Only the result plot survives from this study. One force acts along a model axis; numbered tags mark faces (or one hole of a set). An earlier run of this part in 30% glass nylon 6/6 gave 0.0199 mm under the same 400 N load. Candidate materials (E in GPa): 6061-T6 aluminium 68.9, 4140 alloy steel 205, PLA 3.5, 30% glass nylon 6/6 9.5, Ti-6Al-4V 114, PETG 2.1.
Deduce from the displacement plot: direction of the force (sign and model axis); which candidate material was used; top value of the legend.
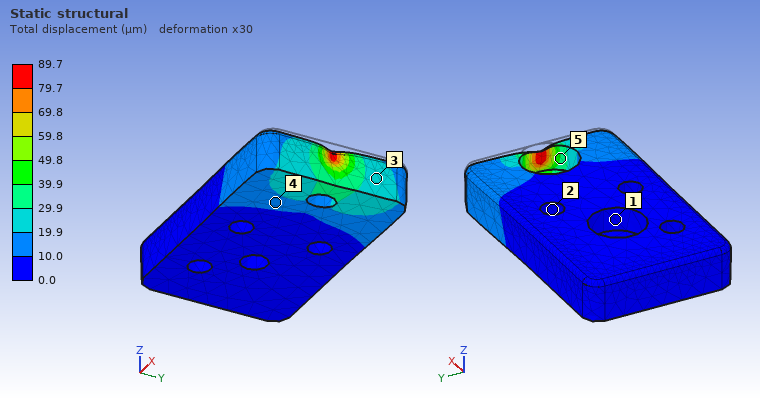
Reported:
-X
PETG
89.7 µm
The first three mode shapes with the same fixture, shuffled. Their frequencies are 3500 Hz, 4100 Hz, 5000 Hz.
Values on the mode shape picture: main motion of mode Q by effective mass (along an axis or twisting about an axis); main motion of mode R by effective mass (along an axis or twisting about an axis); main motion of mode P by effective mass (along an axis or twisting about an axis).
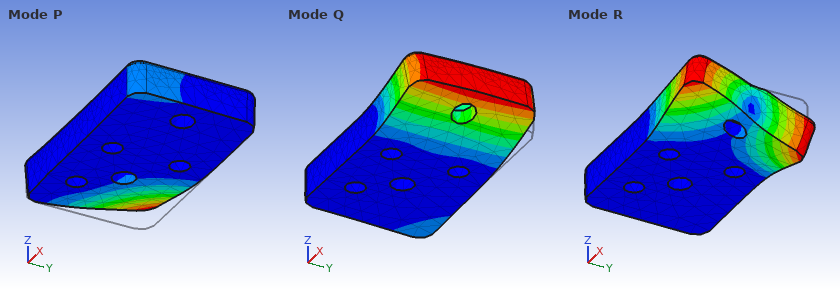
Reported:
along Z
twisting about X
along Z
